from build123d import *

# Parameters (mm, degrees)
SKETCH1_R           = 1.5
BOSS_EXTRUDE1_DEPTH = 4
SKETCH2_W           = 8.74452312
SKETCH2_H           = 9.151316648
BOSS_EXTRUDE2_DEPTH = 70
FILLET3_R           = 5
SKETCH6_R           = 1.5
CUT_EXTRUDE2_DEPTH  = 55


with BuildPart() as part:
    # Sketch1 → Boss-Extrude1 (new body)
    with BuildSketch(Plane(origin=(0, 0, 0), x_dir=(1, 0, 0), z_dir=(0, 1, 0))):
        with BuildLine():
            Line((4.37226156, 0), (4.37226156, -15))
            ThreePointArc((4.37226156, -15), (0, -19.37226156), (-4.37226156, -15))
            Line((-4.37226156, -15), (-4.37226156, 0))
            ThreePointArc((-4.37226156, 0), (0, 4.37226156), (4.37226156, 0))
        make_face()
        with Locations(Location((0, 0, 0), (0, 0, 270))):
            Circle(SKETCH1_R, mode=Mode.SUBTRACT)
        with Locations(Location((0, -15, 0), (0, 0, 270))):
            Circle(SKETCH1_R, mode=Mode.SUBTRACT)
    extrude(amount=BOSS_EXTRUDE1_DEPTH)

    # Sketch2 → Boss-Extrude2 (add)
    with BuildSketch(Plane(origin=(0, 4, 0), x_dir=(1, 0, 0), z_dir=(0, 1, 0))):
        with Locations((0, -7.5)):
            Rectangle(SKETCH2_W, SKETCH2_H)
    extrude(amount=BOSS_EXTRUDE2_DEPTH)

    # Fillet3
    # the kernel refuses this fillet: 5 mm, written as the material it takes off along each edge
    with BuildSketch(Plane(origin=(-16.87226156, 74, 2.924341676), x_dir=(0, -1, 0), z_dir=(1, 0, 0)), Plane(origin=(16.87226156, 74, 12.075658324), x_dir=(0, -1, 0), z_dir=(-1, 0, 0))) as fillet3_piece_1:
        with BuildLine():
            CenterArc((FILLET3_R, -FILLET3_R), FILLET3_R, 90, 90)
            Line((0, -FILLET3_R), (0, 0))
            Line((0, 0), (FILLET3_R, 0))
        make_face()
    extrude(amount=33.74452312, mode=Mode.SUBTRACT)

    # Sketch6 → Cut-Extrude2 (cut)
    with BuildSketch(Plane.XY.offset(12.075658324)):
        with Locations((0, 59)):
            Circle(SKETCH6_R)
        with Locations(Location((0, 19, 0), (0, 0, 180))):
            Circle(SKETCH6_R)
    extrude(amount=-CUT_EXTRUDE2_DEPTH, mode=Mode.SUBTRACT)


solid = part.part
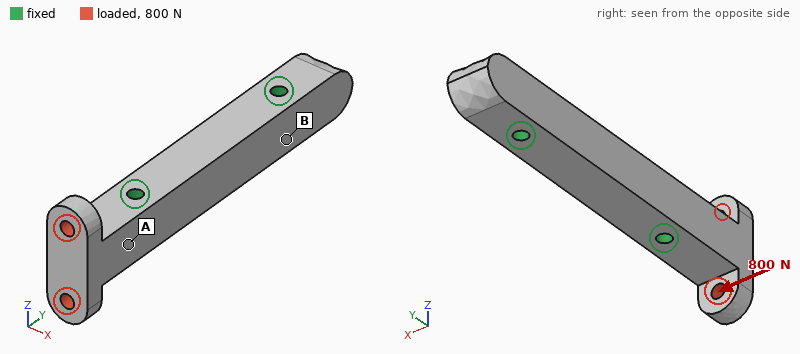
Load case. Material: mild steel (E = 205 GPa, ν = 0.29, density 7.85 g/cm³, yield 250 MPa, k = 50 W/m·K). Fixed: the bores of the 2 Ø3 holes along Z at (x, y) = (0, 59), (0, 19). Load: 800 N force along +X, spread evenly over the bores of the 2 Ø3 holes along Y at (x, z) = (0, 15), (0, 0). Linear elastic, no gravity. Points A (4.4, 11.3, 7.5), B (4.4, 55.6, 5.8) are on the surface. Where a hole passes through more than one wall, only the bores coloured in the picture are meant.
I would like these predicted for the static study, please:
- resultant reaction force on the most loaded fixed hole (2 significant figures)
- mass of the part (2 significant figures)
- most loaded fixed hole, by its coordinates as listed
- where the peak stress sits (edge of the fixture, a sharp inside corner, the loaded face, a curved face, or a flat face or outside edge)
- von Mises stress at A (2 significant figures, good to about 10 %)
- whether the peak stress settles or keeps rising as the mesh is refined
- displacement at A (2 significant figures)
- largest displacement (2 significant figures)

910 N
48 g
(0, 19)
edge of the fixture
64 MPa
keeps rising
8.5 µm
26 µm
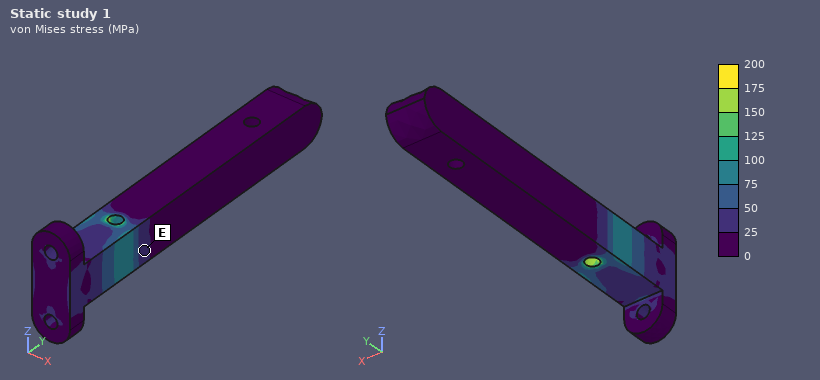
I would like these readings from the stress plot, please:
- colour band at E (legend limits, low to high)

25 to 50 MPa
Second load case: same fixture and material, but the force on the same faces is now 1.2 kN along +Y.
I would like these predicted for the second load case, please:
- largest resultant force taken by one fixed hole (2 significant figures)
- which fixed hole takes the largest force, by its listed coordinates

1.2 kN
(0, 19)
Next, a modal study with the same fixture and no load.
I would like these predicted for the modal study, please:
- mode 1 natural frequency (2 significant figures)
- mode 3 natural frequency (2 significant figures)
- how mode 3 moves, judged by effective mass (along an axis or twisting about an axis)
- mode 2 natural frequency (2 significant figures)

11 kHz
19 kHz
twisting about Y
13 kHz
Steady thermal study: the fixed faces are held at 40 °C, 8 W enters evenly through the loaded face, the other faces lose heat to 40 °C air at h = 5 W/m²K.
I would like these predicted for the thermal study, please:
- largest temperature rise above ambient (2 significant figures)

45 K
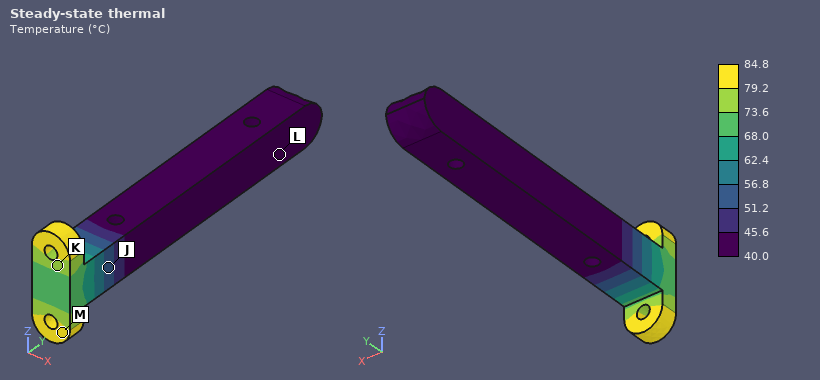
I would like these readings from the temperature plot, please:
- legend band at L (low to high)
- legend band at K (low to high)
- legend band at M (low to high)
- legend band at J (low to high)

40.0 to 45.6 °C
73.6 to 79.2 °C
79.2 to 84.8 °C
51.2 to 56.8 °C
